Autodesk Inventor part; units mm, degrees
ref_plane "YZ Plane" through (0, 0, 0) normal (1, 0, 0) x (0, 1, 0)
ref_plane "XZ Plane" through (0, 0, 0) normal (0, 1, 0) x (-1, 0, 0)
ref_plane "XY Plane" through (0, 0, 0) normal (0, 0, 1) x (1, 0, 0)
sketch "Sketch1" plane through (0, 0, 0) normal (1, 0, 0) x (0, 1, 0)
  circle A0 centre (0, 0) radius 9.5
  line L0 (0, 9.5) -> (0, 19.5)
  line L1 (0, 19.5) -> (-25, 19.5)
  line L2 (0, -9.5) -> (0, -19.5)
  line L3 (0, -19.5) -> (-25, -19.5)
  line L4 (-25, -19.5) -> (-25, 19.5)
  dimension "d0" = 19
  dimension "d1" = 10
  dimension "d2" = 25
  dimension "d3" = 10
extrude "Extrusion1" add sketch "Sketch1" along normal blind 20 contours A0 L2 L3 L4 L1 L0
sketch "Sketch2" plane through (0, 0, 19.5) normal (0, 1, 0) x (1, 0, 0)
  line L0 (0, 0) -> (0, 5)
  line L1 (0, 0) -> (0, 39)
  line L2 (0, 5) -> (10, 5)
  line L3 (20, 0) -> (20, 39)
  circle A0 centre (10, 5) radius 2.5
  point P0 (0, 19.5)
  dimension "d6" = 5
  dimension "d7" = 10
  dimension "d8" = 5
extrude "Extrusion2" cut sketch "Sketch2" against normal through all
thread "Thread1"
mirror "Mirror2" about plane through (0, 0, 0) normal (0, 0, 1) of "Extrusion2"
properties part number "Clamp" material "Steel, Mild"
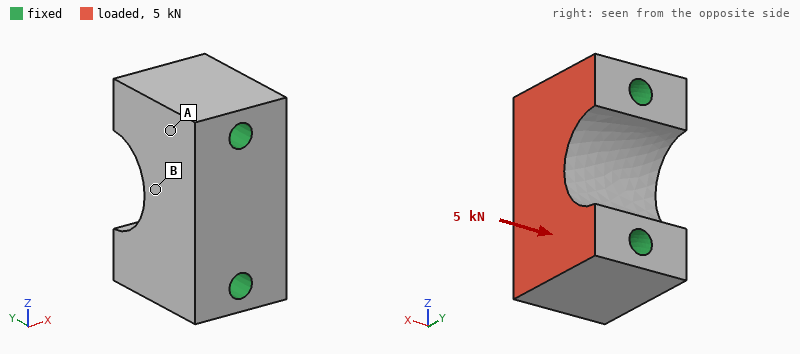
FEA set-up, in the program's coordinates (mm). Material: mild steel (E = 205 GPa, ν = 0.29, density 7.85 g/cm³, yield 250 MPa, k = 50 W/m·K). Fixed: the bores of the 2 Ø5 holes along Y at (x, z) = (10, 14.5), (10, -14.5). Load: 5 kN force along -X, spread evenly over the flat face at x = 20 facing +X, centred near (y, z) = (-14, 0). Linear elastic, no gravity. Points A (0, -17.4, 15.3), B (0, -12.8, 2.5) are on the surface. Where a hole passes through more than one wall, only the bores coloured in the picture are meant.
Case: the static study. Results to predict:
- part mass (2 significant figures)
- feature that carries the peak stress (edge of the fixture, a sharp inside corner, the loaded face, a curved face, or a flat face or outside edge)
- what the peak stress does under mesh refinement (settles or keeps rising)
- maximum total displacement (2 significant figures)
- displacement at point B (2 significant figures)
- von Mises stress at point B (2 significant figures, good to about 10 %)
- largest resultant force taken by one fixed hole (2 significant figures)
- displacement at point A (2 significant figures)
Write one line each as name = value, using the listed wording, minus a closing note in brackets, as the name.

part mass = 120 g
feature that carries the peak stress = edge of the fixture
what the peak stress does under mesh refinement = keeps rising
maximum total displacement = 0.86 µm
displacement at point B = 0.40 µm
von Mises stress at point B = 5.4 MPa
largest resultant force taken by one fixed hole = 2.5 kN
displacement at point A = 0.19 µm
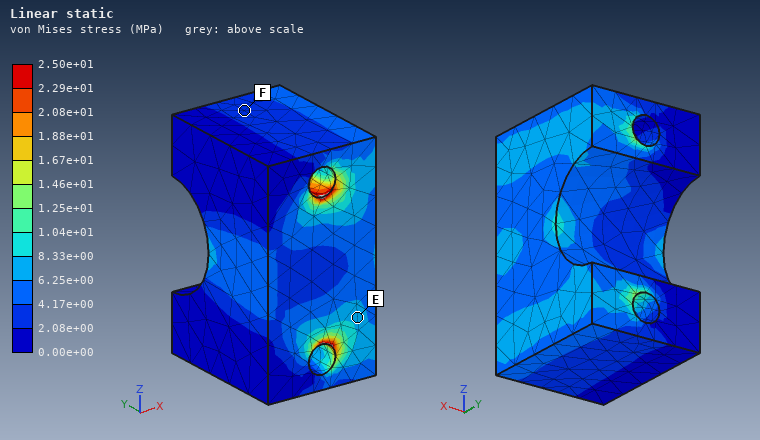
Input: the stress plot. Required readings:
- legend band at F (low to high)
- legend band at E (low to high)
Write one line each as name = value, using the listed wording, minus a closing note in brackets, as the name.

legend band at F = 2.08e+00 to 4.17e+00 MPa
legend band at E = 6.25e+00 to 8.33e+00 MPa
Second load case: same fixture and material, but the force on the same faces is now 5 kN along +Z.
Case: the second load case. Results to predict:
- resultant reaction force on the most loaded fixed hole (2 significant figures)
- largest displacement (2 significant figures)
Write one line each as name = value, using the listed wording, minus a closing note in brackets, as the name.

resultant reaction force on the most loaded fixed hole = 2.8 kN
largest displacement = 1.7 µm
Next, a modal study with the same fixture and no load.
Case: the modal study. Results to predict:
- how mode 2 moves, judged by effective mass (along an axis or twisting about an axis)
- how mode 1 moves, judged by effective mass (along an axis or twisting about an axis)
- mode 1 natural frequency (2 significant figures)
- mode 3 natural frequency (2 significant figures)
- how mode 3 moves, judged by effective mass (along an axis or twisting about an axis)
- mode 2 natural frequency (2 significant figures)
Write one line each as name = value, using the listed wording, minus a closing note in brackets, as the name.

how mode 2 moves, judged by effective mass = along Y
how mode 1 moves, judged by effective mass = along X
mode 1 natural frequency = 43 kHz
mode 3 natural frequency = 57 kHz
how mode 3 moves, judged by effective mass = twisting about Z
mode 2 natural frequency = 49 kHz
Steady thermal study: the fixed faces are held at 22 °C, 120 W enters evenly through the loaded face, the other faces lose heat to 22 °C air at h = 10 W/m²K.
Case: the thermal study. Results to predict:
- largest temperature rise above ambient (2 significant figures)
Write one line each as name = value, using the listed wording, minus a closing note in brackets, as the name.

largest temperature rise above ambient = 37 K
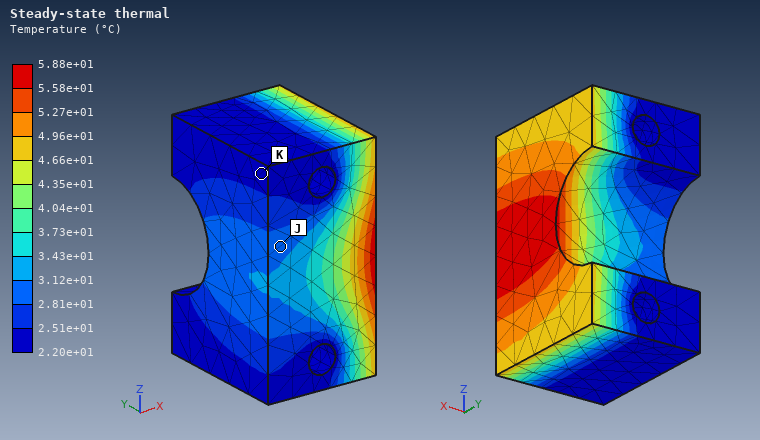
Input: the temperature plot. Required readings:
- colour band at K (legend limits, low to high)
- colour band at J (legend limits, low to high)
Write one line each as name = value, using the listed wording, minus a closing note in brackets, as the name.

colour band at K = 2.20e+01 to 2.51e+01 °C
colour band at J = 2.81e+01 to 3.12e+01 °C
